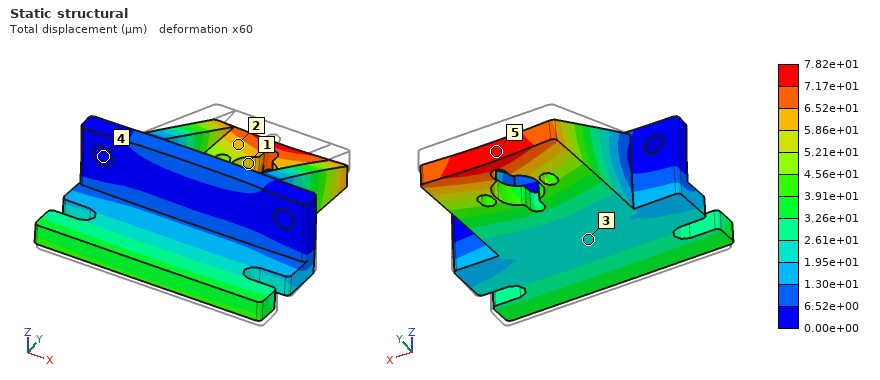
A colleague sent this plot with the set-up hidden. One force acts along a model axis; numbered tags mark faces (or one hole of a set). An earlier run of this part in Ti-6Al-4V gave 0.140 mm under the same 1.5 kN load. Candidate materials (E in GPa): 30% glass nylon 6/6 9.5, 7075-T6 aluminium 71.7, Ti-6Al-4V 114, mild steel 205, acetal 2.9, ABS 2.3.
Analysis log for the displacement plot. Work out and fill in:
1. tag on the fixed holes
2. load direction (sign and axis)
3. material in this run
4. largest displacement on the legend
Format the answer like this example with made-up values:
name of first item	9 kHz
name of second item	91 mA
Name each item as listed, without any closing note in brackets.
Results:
tag on the fixed holes	4
load direction	-Z
material in this run	mild steel
largest displacement on the legend	7.82e+01 µm
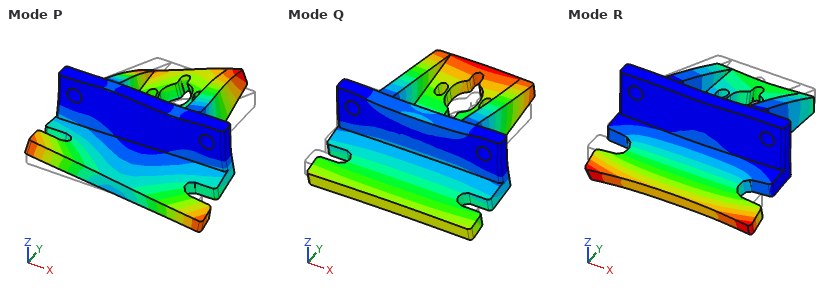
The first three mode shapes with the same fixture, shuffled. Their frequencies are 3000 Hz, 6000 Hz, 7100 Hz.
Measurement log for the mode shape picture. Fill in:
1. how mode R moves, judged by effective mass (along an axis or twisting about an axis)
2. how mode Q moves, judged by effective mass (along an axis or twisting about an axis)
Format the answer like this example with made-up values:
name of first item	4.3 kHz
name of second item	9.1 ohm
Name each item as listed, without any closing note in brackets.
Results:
how mode R moves, judged by effective mass	along Z
how mode Q moves, judged by effective mass	along Y
